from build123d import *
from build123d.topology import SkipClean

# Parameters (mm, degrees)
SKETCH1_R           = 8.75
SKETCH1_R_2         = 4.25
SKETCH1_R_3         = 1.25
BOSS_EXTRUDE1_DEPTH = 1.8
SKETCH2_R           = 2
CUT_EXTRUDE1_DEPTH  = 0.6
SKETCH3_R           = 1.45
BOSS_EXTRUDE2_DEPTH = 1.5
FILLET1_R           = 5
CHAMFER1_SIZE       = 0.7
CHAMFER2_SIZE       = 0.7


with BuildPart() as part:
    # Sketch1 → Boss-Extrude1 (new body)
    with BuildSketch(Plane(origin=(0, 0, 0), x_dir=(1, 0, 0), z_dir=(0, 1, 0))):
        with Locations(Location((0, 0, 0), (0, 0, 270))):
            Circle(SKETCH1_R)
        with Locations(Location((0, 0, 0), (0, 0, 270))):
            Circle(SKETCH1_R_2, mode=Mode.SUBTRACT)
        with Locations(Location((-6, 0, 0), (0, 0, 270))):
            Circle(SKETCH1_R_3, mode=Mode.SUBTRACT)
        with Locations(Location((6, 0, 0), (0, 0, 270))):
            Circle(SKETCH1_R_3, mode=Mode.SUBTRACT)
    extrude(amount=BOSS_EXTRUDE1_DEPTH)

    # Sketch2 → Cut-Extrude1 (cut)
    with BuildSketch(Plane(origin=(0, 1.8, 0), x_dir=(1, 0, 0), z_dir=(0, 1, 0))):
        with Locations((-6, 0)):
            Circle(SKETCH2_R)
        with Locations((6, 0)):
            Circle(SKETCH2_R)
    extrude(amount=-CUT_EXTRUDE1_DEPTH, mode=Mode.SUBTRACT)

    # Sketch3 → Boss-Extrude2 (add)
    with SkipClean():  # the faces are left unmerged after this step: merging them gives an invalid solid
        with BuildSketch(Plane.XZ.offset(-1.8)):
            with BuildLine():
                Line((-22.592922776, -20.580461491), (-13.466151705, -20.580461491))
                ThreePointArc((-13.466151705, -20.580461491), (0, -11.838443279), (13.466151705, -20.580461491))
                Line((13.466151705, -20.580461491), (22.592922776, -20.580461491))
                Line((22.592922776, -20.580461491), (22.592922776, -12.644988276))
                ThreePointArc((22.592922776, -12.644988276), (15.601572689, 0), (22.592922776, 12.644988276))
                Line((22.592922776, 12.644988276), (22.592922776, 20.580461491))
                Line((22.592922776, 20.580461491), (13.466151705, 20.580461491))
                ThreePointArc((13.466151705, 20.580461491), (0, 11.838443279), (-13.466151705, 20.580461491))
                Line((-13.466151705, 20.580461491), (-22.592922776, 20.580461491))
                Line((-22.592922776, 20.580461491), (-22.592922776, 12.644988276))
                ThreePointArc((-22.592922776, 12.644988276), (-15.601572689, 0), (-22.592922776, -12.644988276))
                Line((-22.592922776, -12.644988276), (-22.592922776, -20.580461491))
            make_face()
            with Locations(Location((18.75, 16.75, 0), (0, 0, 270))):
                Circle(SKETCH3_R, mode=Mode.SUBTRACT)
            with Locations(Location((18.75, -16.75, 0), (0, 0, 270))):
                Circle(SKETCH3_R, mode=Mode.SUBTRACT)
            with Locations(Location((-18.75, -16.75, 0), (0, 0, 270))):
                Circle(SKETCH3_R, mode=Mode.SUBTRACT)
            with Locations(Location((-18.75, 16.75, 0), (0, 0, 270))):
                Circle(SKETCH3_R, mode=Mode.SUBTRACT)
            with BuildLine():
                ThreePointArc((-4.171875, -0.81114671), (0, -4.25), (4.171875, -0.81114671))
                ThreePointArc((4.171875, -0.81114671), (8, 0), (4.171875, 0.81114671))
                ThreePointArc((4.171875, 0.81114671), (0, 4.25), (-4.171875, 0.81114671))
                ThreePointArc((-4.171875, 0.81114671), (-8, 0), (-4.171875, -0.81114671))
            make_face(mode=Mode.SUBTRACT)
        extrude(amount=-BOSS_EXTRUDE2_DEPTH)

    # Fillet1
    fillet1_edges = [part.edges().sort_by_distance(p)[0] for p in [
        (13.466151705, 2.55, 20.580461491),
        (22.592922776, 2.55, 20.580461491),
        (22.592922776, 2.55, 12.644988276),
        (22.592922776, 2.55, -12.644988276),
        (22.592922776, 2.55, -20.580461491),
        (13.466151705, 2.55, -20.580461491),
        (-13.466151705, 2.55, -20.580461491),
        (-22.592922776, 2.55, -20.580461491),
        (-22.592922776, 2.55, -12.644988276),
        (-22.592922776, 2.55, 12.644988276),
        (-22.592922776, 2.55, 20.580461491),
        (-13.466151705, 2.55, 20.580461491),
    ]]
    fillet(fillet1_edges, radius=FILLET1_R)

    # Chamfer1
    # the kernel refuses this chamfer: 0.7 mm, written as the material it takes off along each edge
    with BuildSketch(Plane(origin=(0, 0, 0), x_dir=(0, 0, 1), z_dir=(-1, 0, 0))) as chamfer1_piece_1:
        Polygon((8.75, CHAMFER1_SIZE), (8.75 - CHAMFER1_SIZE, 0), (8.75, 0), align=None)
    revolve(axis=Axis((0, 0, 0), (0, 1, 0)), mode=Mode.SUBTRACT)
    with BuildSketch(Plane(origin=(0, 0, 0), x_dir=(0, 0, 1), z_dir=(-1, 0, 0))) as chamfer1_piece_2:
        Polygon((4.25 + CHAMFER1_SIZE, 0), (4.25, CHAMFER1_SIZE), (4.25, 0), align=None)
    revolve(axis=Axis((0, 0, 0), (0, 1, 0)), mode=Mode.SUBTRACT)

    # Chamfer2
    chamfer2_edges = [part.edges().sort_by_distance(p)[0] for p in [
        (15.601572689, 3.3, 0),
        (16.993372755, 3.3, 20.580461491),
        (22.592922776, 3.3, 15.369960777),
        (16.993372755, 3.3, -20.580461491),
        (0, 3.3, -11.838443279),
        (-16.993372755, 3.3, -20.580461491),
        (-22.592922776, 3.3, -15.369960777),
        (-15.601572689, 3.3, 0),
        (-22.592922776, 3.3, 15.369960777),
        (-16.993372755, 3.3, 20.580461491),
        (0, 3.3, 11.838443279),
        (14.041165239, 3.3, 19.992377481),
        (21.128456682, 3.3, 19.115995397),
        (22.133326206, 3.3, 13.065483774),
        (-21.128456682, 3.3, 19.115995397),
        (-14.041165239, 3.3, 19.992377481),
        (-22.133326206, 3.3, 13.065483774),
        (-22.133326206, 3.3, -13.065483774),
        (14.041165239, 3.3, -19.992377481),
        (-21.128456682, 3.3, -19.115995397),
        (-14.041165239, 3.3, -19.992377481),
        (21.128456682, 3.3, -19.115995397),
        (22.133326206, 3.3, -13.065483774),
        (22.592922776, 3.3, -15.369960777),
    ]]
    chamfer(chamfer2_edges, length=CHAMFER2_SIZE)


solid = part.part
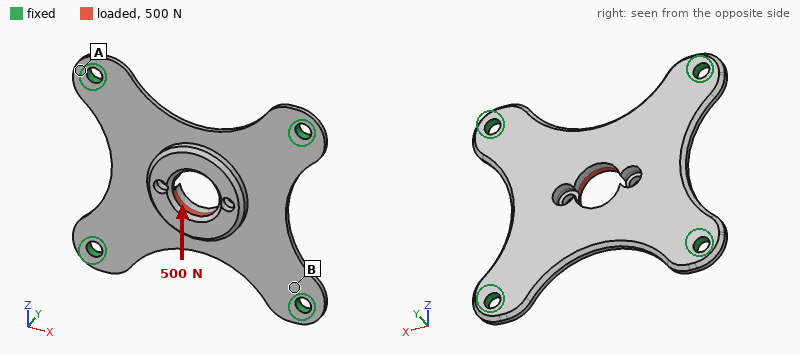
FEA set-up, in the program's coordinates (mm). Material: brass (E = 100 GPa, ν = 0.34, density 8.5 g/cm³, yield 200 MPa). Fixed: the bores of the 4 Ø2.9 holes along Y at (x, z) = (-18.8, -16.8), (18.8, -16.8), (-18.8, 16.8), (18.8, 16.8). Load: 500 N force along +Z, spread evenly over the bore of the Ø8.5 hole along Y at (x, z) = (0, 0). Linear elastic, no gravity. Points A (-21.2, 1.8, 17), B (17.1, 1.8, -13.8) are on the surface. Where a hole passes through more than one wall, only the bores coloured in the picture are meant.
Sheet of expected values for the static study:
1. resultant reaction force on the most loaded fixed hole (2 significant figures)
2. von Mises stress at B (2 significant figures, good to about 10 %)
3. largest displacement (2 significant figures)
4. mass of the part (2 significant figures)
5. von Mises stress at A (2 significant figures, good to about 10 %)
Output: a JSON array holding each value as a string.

["160 N", "16 MPa", "15 µm", "16 g", "6.0 MPa"]
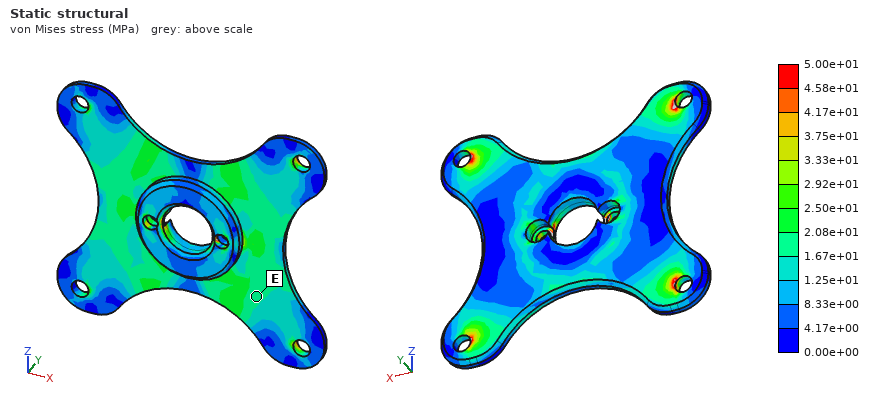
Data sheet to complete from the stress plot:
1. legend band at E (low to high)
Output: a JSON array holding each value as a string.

["1.67e+01 to 2.08e+01 MPa"]
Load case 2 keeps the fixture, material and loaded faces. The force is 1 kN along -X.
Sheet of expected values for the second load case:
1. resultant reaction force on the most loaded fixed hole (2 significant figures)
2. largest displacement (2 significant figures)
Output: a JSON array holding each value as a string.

["310 N", "20 µm"]
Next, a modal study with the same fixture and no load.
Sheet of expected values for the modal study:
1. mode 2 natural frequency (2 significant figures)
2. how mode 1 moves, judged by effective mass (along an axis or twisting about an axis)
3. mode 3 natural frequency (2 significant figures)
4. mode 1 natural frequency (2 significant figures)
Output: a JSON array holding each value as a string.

["5700 Hz", "along Y", "5800 Hz", "3000 Hz"]
